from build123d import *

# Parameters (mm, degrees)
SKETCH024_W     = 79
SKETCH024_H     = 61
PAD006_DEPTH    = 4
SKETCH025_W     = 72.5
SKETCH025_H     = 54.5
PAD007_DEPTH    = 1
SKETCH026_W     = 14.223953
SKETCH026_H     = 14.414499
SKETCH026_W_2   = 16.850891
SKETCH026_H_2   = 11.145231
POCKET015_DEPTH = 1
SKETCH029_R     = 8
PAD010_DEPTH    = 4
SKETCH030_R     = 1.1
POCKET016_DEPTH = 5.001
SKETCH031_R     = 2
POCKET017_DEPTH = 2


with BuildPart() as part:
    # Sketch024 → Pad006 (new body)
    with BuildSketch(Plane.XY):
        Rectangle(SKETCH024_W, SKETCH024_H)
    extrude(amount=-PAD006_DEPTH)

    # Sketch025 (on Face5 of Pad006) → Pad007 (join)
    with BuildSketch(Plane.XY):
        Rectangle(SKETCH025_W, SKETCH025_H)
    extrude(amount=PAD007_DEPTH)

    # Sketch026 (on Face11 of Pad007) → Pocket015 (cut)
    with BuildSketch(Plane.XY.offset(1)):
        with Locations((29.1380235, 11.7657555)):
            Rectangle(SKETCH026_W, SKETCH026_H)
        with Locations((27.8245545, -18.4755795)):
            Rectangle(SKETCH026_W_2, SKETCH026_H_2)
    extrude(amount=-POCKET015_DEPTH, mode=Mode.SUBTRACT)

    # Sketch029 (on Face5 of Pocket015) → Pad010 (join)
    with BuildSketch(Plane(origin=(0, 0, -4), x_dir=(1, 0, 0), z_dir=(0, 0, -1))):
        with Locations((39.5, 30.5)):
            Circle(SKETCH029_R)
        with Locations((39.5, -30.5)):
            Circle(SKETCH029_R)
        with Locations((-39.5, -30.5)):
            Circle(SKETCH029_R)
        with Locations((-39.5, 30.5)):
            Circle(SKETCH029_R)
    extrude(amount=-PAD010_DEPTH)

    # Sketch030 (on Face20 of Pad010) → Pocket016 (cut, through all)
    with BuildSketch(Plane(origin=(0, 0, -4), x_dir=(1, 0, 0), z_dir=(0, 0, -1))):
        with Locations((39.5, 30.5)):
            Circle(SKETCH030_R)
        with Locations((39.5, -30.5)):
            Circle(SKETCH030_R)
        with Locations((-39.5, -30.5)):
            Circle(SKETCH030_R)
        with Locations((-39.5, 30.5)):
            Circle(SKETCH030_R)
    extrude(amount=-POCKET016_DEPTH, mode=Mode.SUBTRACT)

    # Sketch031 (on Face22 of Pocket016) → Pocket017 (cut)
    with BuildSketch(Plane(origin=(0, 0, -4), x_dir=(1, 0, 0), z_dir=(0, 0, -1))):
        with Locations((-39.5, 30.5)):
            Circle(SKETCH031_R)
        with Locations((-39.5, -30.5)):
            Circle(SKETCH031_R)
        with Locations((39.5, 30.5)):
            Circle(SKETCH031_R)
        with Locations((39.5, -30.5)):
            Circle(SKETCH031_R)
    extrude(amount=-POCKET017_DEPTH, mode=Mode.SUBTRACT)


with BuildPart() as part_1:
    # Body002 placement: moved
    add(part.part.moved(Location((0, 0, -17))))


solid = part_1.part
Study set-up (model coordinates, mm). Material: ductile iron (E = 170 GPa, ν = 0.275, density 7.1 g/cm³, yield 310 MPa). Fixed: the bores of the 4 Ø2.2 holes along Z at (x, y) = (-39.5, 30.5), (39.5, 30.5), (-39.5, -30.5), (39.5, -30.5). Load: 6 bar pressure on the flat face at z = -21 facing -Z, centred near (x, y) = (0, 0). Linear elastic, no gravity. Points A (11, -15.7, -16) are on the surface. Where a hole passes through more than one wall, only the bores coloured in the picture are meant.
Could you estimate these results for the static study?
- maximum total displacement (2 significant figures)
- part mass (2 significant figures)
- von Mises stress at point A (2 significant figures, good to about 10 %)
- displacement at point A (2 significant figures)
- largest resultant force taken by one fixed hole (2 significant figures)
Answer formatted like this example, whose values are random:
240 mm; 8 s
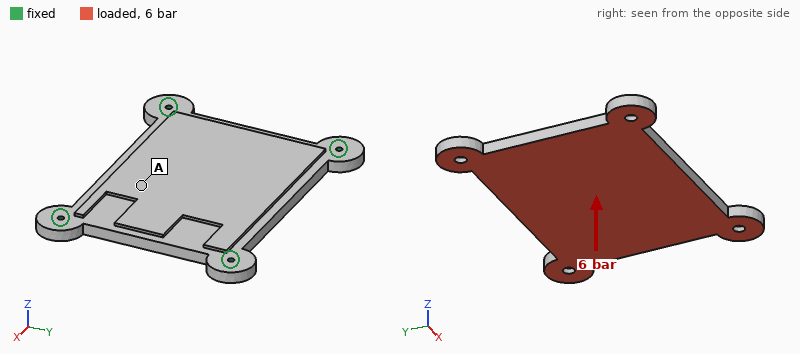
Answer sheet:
0.14 mm; 180 g; 60 MPa; 0.13 mm; 1.1 kN
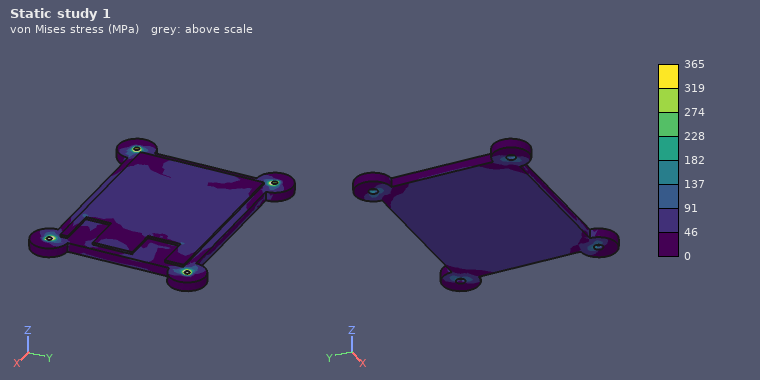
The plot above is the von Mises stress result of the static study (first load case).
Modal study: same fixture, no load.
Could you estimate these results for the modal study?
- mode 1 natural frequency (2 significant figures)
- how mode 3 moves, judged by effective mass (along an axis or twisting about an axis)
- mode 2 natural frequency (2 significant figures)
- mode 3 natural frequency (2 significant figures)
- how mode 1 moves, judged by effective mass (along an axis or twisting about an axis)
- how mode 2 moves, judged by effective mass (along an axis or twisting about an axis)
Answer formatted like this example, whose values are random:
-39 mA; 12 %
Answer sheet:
2000 Hz; twisting about Y; 3900 Hz; 4500 Hz; along Z; twisting about X
